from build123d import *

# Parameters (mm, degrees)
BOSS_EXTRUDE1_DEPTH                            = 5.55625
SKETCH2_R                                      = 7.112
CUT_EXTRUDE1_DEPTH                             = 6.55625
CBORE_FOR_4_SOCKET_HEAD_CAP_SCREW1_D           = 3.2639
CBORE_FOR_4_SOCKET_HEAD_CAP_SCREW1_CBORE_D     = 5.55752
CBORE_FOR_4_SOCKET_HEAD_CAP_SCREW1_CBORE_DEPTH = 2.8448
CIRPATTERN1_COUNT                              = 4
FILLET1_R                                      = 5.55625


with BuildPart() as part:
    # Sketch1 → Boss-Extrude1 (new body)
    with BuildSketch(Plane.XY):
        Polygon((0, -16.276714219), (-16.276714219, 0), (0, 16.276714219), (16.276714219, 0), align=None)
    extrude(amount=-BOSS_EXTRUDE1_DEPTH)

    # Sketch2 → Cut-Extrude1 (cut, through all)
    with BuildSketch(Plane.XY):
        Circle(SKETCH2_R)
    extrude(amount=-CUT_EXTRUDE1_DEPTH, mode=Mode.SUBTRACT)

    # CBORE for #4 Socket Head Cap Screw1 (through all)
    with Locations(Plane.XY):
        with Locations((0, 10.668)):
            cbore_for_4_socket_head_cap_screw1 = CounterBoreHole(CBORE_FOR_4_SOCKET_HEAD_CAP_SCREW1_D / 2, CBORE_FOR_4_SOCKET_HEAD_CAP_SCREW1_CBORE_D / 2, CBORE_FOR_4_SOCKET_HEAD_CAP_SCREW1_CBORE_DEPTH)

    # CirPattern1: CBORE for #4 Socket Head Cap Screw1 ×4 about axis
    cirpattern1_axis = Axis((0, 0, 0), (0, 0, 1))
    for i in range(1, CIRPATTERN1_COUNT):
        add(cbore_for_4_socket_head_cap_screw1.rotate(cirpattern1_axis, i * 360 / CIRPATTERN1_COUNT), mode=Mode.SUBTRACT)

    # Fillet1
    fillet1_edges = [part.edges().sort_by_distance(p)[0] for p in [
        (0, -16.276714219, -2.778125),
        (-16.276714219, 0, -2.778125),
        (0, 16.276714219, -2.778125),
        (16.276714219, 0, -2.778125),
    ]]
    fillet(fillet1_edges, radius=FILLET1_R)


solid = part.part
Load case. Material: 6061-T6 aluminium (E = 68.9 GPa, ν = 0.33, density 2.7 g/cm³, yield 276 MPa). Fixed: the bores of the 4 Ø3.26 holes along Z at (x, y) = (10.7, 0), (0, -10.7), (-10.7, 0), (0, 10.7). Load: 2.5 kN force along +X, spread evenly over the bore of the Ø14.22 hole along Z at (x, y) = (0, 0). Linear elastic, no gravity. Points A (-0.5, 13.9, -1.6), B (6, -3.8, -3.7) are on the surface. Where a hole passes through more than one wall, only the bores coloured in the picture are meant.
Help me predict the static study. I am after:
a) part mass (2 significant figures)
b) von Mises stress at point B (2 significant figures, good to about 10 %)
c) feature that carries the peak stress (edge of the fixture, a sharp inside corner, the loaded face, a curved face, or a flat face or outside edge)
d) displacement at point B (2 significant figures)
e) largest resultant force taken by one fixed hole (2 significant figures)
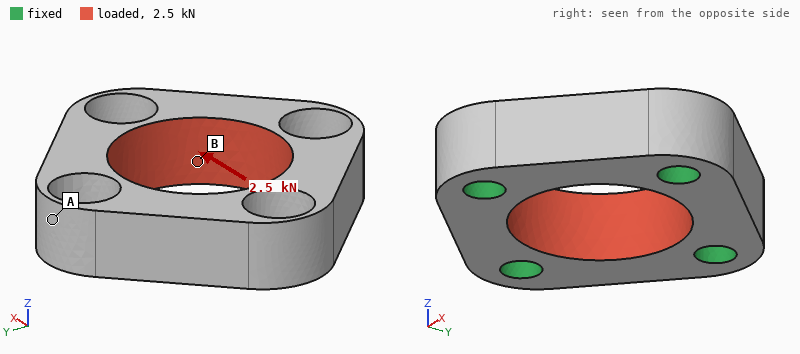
4.2 g
21 MPa
edge of the fixture
2.8 µm
630 N
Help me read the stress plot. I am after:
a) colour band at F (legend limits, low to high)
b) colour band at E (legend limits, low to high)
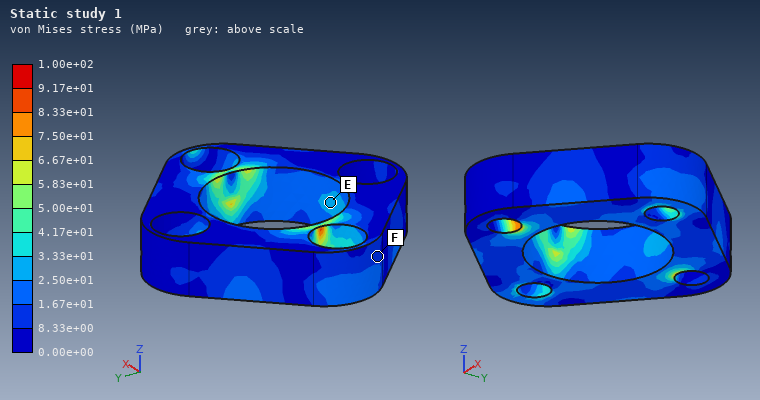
8.33e+00 to 1.67e+01 MPa
2.50e+01 to 3.33e+01 MPa
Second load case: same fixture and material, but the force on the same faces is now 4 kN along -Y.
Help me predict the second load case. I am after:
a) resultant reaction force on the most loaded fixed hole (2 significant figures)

1.0 kN
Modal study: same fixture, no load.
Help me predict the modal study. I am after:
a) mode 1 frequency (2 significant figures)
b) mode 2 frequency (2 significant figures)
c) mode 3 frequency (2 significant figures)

54 kHz
62 kHz
62 kHz
